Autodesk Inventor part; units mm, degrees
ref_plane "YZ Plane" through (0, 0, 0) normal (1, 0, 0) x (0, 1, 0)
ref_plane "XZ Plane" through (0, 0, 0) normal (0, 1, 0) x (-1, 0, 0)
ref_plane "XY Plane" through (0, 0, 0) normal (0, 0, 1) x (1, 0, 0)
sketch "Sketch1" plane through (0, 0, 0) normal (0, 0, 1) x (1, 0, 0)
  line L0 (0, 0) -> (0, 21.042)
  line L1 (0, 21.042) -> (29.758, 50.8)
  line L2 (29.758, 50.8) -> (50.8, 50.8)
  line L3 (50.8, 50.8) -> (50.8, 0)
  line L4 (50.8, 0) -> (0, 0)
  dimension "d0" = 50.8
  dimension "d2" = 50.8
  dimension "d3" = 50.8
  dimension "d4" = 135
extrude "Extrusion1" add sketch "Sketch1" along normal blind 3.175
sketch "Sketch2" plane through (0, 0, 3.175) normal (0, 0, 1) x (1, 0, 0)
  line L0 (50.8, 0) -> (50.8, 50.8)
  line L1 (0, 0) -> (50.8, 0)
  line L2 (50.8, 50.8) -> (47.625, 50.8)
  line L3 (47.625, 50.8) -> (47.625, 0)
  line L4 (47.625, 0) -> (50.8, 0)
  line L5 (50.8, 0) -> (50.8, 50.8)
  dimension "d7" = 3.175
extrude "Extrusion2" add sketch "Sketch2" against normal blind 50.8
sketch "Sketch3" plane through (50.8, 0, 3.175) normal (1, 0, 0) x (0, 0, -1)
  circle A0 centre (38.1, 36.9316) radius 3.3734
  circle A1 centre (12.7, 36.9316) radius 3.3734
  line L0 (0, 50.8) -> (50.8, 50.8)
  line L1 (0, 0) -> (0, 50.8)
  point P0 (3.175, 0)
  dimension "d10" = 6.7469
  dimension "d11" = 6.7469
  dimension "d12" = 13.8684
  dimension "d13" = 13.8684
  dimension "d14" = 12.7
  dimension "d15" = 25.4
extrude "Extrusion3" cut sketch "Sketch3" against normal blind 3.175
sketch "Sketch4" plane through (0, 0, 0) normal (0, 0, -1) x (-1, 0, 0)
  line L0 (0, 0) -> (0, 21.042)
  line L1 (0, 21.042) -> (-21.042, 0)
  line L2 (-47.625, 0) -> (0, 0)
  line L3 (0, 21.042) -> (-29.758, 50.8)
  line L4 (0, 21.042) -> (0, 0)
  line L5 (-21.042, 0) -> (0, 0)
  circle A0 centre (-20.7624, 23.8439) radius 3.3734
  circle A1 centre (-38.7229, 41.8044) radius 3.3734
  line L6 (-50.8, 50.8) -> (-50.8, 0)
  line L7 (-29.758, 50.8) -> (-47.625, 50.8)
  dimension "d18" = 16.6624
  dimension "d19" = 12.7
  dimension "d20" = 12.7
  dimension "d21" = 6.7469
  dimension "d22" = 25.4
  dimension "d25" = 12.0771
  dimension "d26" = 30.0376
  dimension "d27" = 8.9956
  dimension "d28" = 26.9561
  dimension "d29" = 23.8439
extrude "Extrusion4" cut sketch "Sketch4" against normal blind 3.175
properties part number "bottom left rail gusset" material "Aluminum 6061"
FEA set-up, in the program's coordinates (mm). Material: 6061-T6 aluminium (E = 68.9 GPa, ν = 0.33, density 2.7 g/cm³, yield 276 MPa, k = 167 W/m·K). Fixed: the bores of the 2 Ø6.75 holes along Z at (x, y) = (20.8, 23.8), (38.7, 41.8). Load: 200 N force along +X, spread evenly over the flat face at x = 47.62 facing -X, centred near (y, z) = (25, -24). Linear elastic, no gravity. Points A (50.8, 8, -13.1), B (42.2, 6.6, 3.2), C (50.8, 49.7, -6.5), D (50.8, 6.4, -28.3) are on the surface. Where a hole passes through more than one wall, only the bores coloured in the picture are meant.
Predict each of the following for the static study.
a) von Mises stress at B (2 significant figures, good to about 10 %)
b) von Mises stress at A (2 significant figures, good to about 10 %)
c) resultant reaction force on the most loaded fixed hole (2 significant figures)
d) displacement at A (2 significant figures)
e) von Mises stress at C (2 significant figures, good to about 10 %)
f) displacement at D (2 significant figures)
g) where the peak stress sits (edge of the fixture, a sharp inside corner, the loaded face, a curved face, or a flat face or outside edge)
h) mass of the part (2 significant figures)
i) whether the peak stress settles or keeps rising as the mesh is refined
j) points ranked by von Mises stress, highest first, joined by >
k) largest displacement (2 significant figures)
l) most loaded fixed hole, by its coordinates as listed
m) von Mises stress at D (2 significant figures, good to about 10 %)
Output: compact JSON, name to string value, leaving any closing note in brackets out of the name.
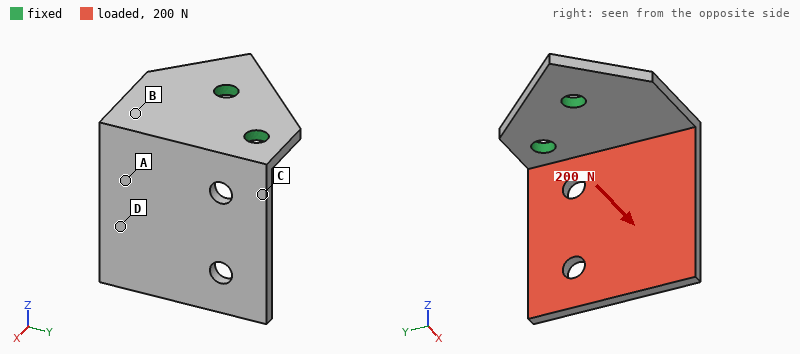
{"von Mises stress at B": "39 MPa", "von Mises stress at A": "26 MPa", "resultant reaction force on the most loaded fixed hole": "170 N", "displacement at A": "0.19 mm", "von Mises stress at C": "52 MPa", "displacement at D": "0.38 mm", "where the peak stress sits": "edge of the fixture", "mass of the part": "36 g", "whether the peak stress settles or keeps rising as the mesh is refined": "keeps rising", "points ranked by von Mises stress, highest first, joined by >": "C > B > A > D", "largest displacement": "0.67 mm", "most loaded fixed hole, by its coordinates as listed": "(20.8, 23.8)", "von Mises stress at D": "9.4 MPa"}
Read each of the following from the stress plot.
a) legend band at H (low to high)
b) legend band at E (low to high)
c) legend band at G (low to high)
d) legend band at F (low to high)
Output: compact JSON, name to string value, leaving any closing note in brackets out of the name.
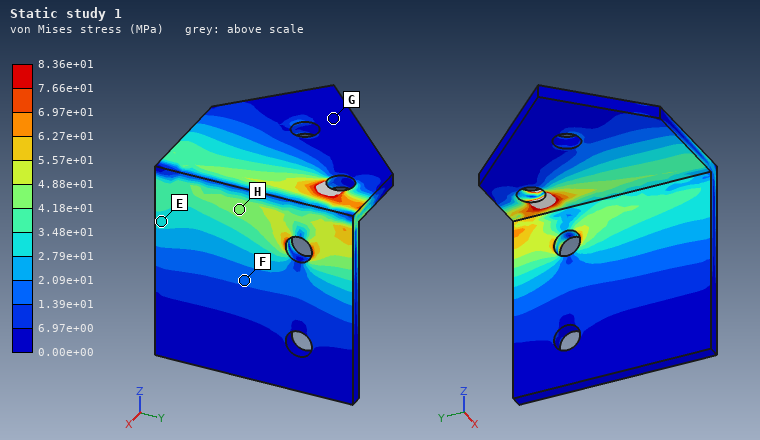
{"legend band at H": "4.18e+01 to 4.88e+01 MPa", "legend band at E": "2.79e+01 to 3.48e+01 MPa", "legend band at G": "0.00e+00 to 6.97e+00 MPa", "legend band at F": "1.39e+01 to 2.09e+01 MPa"}
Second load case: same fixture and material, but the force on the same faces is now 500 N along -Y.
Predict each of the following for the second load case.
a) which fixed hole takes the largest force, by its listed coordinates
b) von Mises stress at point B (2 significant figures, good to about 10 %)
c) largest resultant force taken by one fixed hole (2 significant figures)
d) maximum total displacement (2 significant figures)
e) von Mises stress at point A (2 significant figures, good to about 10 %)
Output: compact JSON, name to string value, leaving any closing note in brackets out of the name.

{"which fixed hole takes the largest force, by its listed coordinates": "(38.7, 41.8)", "von Mises stress at point B": "20 MPa", "largest resultant force taken by one fixed hole": "530 N", "maximum total displacement": "0.59 mm", "von Mises stress at point A": "18 MPa"}
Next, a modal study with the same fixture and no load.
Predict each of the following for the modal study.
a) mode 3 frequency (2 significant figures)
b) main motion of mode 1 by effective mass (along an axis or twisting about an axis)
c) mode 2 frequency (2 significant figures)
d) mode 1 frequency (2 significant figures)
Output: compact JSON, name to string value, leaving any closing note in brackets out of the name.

{"mode 3 frequency": "2300 Hz", "main motion of mode 1 by effective mass": "along X", "mode 2 frequency": "1400 Hz", "mode 1 frequency": "750 Hz"}
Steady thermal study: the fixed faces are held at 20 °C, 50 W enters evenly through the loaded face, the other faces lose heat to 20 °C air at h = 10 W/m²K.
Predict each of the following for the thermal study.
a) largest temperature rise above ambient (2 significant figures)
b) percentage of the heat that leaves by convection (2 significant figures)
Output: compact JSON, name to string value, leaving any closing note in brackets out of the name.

{"largest temperature rise above ambient": "78 K", "percentage of the heat that leaves by convection": "4.8 %"}
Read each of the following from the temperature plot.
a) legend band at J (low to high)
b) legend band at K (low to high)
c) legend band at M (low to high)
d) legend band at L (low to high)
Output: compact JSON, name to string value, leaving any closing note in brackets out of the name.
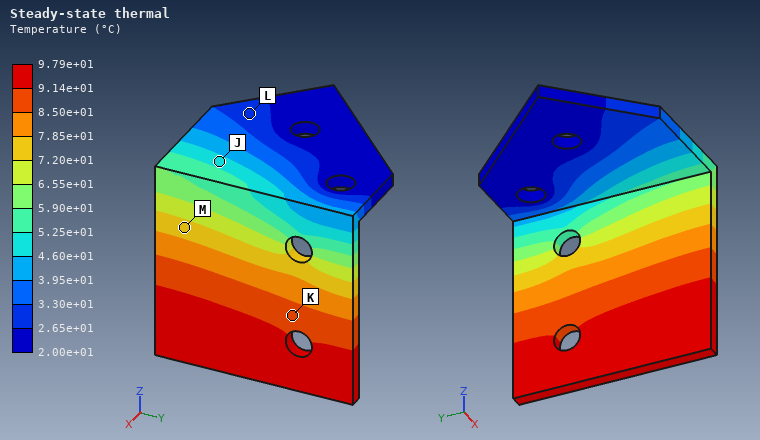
{"legend band at J": "4.60e+01 to 5.25e+01 °C", "legend band at K": "8.50e+01 to 9.14e+01 °C", "legend band at M": "7.20e+01 to 7.85e+01 °C", "legend band at L": "2.65e+01 to 3.30e+01 °C"}
